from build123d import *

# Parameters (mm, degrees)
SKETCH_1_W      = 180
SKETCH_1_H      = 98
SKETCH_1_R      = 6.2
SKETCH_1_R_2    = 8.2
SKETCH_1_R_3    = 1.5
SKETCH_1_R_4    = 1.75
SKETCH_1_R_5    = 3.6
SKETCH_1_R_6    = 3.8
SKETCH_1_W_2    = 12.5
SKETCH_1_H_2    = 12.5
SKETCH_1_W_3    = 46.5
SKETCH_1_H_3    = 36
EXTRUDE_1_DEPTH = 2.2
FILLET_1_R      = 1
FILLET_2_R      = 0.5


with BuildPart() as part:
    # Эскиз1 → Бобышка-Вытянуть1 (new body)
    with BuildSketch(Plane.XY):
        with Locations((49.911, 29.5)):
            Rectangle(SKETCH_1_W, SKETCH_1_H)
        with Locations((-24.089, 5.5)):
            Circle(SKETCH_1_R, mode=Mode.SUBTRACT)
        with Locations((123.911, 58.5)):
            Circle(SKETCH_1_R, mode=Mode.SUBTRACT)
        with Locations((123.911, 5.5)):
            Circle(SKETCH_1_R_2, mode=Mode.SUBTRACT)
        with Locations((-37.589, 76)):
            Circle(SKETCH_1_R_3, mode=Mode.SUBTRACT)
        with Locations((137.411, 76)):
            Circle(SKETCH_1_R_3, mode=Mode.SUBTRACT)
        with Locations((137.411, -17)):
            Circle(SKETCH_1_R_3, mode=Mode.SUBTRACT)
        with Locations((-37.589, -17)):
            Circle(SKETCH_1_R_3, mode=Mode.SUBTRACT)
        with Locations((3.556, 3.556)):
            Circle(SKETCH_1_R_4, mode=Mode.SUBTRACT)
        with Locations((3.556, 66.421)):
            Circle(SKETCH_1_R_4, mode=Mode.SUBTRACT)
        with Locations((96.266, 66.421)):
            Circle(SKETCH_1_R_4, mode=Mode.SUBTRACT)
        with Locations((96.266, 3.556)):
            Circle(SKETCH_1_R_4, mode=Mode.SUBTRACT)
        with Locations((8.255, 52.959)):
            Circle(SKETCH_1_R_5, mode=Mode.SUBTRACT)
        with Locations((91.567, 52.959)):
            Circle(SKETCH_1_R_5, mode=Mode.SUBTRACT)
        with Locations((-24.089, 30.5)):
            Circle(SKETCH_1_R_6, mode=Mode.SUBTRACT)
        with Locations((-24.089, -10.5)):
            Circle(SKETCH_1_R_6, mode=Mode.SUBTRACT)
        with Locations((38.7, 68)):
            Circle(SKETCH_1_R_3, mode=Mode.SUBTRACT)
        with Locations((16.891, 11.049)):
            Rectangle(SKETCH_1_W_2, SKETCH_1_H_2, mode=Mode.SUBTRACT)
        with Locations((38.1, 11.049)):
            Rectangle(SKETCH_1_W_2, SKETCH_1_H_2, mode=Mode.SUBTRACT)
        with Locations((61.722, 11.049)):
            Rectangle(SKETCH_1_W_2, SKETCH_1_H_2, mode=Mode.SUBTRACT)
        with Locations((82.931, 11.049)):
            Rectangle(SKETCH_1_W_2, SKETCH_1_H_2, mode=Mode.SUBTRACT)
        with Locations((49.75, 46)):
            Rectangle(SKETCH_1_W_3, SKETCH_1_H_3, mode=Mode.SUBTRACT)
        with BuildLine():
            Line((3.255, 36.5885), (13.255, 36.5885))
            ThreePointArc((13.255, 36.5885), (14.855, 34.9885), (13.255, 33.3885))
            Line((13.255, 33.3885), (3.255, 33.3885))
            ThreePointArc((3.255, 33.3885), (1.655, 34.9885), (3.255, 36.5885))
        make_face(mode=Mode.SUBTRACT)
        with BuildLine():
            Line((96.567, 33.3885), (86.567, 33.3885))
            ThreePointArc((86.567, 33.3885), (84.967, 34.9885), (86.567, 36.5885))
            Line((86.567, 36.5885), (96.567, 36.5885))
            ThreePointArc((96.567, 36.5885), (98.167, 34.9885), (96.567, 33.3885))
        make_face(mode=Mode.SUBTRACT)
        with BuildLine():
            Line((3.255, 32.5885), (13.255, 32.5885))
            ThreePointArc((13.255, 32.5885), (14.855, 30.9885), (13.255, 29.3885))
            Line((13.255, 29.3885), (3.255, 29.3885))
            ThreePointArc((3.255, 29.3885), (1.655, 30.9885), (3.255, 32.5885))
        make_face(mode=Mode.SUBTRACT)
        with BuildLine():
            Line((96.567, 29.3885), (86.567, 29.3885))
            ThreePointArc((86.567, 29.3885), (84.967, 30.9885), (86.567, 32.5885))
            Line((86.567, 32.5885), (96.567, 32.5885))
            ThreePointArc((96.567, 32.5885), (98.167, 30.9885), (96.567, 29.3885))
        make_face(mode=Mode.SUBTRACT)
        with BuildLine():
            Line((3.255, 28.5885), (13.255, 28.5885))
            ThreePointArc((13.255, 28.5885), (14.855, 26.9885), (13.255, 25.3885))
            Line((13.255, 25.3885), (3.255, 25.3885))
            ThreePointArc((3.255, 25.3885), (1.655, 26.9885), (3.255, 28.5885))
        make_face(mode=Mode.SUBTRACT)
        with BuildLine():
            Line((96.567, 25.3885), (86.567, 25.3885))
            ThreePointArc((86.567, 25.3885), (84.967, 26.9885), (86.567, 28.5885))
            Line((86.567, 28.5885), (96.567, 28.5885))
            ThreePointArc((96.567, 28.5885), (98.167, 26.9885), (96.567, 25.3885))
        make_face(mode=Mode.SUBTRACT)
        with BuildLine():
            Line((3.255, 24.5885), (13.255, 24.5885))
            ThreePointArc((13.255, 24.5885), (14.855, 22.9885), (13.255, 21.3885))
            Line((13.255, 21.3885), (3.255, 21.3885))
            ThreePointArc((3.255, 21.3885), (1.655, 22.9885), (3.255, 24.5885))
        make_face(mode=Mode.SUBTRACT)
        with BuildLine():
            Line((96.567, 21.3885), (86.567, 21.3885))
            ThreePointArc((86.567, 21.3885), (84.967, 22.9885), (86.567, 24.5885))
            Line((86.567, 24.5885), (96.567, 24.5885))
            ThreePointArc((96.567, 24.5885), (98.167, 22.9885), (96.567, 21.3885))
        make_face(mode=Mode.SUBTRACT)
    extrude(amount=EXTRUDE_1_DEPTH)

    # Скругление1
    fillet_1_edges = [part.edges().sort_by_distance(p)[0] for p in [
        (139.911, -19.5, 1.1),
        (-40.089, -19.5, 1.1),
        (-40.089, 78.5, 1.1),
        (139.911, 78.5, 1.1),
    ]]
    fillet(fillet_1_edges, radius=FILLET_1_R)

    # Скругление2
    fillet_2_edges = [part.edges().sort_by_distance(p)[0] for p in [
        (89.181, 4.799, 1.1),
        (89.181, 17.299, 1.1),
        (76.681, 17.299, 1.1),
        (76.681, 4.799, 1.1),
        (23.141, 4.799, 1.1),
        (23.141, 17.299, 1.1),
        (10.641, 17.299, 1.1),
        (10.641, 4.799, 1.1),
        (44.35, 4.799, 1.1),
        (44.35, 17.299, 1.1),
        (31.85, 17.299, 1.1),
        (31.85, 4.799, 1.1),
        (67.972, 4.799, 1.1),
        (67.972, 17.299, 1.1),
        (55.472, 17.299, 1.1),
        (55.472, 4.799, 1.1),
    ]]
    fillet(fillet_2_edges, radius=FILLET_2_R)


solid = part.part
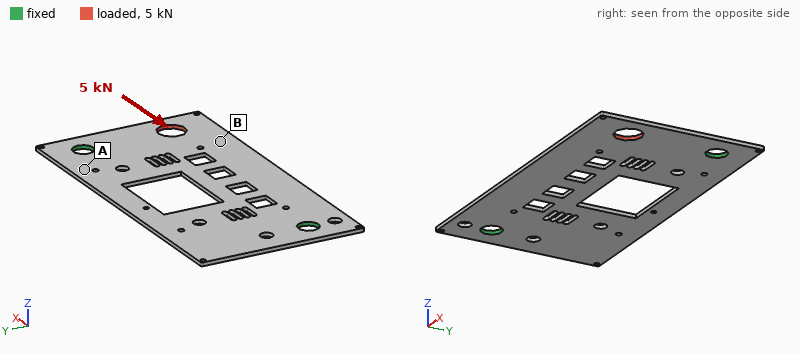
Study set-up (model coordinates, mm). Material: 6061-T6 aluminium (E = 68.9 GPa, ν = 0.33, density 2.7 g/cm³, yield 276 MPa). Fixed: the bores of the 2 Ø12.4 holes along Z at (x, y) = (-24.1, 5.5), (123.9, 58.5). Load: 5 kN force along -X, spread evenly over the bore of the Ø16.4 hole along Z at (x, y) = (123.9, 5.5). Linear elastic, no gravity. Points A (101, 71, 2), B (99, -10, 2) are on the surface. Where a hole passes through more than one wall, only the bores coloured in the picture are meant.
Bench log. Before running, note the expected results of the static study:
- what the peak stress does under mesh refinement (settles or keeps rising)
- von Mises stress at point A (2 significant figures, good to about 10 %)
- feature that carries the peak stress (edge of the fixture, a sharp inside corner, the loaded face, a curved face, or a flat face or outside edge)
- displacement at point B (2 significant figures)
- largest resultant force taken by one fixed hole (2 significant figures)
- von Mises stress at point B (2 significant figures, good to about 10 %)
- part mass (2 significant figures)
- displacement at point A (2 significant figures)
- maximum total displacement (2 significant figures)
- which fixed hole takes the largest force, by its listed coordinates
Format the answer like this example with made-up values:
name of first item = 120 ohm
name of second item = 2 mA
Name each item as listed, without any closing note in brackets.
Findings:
what the peak stress does under mesh refinement = keeps rising
von Mises stress at point A = 18 MPa
feature that carries the peak stress = a sharp inside corner
displacement at point B = 0.084 mm
largest resultant force taken by one fixed hole = 2.9 kN
von Mises stress at point B = 55 MPa
part mass = 85 g
displacement at point A = 0.018 mm
maximum total displacement = 0.11 mm
which fixed hole takes the largest force, by its listed coordinates = (-24.1, 5.5)
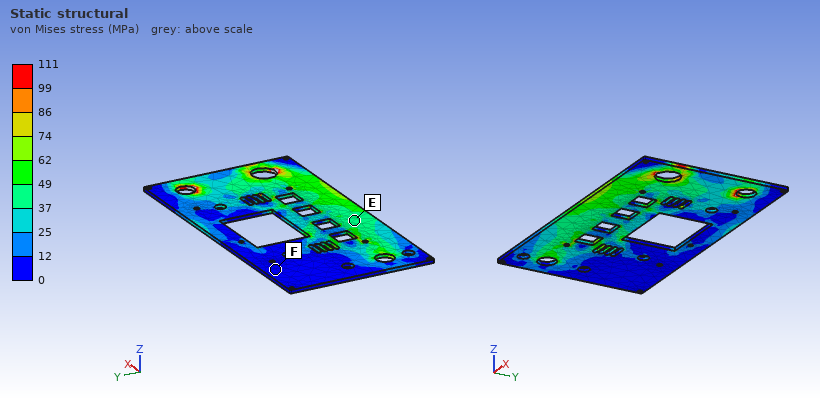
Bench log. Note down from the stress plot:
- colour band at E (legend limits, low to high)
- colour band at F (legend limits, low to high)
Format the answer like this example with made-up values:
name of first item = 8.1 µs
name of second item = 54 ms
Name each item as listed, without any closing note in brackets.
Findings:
colour band at E = 37 to 49 MPa
colour band at F = 0 to 12 MPa
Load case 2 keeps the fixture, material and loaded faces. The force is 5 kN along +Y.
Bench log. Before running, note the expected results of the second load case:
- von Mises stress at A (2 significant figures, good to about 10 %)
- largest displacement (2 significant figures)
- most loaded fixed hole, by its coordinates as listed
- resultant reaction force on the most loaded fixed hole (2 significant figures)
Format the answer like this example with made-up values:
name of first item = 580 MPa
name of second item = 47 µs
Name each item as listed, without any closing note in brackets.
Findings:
von Mises stress at A = 10 MPa
largest displacement = 69 µm
most loaded fixed hole, by its coordinates as listed = (123.9, 58.5)
resultant reaction force on the most loaded fixed hole = 5.0 kN
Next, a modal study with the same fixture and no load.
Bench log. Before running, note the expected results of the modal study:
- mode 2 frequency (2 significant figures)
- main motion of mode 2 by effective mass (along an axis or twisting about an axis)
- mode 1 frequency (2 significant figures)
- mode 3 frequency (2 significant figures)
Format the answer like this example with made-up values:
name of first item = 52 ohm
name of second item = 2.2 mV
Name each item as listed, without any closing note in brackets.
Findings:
mode 2 frequency = 370 Hz
main motion of mode 2 by effective mass = along Z
mode 1 frequency = 320 Hz
mode 3 frequency = 600 Hz
